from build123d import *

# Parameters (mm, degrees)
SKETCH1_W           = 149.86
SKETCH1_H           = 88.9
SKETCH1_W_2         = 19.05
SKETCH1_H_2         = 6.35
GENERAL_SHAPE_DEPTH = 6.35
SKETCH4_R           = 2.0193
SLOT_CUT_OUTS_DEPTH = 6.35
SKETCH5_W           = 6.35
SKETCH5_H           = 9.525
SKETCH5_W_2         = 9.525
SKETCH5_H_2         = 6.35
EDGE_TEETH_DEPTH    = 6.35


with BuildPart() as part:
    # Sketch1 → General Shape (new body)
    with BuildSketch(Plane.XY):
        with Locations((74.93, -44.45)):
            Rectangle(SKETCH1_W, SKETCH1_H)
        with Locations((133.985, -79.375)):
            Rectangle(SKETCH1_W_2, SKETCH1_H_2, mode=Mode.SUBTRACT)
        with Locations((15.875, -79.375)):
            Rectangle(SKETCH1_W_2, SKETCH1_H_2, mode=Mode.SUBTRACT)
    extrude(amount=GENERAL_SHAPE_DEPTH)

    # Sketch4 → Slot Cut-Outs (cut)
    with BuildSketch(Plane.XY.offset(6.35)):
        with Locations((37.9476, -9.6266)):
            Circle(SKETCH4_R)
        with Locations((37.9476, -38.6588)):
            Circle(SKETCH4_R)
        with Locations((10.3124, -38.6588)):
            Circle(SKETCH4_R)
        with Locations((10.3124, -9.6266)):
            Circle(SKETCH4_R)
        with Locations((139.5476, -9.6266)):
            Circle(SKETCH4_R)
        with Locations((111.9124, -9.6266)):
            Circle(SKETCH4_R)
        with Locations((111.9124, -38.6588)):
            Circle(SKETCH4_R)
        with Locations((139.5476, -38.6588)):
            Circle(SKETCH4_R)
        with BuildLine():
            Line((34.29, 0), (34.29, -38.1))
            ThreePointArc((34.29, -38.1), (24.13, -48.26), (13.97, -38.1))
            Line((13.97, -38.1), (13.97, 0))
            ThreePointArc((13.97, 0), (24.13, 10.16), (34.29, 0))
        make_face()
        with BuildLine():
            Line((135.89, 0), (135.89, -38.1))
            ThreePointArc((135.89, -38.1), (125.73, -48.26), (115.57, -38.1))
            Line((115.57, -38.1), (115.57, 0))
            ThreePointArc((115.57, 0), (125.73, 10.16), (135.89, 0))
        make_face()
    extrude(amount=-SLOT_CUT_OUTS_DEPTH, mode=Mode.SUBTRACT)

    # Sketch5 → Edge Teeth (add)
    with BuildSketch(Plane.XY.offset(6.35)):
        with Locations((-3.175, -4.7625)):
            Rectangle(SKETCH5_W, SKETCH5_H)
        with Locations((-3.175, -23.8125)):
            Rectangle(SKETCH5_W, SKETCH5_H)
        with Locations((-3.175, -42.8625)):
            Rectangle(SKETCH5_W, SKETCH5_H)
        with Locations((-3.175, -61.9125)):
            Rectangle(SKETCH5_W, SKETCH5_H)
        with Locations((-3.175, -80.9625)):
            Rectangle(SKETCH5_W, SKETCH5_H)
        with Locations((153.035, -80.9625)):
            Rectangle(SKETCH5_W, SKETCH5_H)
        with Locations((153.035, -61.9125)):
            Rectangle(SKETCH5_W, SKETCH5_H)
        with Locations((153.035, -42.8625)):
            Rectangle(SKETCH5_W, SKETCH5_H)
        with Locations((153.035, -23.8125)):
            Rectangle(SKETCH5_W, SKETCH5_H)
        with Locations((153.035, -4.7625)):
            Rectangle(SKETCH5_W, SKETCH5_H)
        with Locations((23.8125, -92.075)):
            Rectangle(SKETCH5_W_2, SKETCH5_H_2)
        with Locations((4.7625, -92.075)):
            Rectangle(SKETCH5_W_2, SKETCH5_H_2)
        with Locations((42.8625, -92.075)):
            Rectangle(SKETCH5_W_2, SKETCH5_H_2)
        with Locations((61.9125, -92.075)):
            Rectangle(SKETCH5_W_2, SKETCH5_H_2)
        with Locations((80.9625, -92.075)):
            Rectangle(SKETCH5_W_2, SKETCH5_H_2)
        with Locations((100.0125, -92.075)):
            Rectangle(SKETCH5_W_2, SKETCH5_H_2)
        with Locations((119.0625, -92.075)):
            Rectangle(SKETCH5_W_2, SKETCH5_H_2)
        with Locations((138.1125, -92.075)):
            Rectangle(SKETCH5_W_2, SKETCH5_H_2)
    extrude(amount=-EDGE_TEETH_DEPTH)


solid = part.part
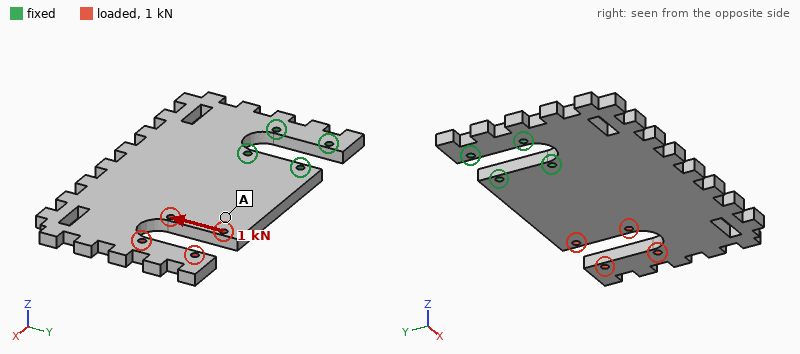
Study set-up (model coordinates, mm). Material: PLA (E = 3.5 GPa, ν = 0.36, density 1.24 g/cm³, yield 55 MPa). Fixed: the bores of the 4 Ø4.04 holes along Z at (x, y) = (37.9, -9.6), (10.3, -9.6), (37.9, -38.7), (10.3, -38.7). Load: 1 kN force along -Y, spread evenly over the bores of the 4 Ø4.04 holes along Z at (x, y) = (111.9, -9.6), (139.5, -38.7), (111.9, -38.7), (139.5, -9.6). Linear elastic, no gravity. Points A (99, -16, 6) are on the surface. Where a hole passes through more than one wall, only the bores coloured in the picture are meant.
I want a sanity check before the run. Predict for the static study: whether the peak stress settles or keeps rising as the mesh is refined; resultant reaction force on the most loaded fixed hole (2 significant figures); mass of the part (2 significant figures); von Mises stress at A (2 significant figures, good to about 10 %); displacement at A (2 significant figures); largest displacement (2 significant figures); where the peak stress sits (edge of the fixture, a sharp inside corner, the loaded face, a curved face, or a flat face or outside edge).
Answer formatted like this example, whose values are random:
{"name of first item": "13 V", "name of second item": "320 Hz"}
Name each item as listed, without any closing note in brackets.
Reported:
{"whether the peak stress settles or keeps rising as the mesh is refined": "keeps rising", "resultant reaction force on the most loaded fixed hole": "2.0 kN", "mass of the part": "96 g", "von Mises stress at A": "3.9 MPa", "displacement at A": "0.52 mm", "largest displacement": "1.2 mm", "where the peak stress sits": "edge of the fixture"}
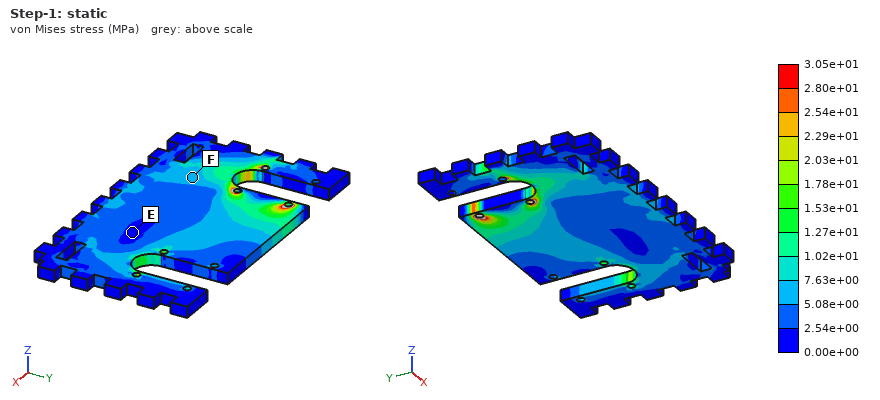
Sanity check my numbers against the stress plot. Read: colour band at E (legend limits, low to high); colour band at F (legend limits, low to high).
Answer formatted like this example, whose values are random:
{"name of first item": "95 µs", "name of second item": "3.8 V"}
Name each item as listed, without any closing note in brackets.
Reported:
{"colour band at E": "0.00e+00 to 2.54e+00 MPa", "colour band at F": "5.08e+00 to 7.63e+00 MPa"}
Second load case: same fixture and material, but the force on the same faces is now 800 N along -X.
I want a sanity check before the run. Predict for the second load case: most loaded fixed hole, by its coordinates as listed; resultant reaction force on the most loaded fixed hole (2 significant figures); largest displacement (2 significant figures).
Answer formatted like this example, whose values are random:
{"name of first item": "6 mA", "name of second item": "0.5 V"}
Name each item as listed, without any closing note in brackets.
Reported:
{"most loaded fixed hole, by its coordinates as listed": "(37.9, -9.6)", "resultant reaction force on the most loaded fixed hole": "420 N", "largest displacement": "2.1 mm"}
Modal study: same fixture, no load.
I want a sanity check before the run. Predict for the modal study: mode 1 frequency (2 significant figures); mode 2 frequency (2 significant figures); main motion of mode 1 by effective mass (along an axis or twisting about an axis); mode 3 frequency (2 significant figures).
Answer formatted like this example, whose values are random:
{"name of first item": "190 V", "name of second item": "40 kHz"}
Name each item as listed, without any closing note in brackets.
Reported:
{"mode 1 frequency": "120 Hz", "mode 2 frequency": "270 Hz", "main motion of mode 1 by effective mass": "along Z", "mode 3 frequency": "520 Hz"}
